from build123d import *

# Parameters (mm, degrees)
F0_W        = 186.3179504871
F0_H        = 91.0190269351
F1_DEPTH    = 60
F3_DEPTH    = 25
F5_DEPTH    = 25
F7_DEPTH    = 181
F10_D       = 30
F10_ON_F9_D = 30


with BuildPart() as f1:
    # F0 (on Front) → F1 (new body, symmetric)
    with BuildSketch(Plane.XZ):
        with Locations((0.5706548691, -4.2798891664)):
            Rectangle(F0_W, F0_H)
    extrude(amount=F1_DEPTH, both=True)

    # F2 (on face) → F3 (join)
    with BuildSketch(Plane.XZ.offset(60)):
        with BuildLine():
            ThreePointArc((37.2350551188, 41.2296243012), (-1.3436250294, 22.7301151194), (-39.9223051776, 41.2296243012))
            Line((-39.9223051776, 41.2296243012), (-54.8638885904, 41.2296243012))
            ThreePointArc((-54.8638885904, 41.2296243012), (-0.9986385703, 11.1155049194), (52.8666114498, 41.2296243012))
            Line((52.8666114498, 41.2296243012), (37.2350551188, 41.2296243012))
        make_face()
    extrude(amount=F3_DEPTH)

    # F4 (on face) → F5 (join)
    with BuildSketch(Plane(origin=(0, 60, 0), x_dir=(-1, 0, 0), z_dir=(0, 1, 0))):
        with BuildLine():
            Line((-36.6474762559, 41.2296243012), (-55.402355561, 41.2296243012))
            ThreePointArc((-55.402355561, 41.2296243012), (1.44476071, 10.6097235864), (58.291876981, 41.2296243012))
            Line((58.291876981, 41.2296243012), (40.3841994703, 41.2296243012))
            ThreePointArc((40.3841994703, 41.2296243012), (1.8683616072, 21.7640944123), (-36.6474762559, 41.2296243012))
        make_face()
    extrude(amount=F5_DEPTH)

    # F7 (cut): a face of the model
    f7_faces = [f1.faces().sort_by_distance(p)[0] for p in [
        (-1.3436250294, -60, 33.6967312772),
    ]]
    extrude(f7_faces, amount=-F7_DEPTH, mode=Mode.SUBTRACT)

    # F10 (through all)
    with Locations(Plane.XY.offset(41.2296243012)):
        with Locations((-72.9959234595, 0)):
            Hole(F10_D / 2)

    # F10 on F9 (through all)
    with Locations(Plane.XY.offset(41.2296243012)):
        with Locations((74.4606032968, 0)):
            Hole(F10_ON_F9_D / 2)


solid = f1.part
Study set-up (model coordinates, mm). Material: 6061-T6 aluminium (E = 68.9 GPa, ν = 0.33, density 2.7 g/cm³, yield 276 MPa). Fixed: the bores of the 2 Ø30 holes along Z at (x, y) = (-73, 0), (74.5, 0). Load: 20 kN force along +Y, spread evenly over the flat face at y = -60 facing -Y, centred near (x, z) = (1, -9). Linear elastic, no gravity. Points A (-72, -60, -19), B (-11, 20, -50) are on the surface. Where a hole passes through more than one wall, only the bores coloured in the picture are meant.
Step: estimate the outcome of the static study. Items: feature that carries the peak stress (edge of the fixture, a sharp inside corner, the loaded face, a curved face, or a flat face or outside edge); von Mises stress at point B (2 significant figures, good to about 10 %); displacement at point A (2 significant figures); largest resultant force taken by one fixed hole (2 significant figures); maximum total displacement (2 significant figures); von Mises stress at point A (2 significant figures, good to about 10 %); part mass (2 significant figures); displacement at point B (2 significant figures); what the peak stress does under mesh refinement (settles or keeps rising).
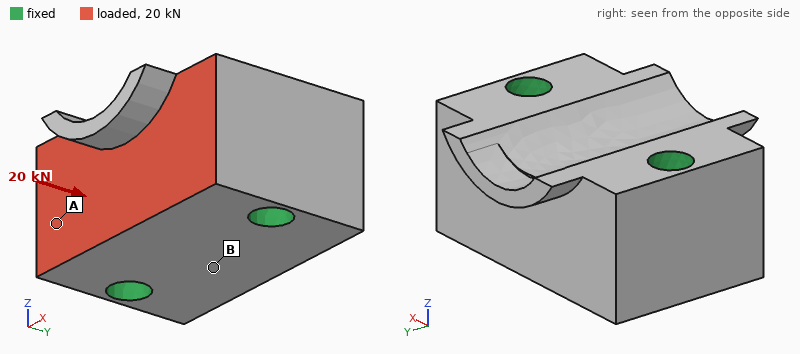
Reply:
edge of the fixture
0.57 MPa
1.1 µm
10 kN
2.6 µm
1.5 MPa
5.0 kg
1.4 µm
keeps rising
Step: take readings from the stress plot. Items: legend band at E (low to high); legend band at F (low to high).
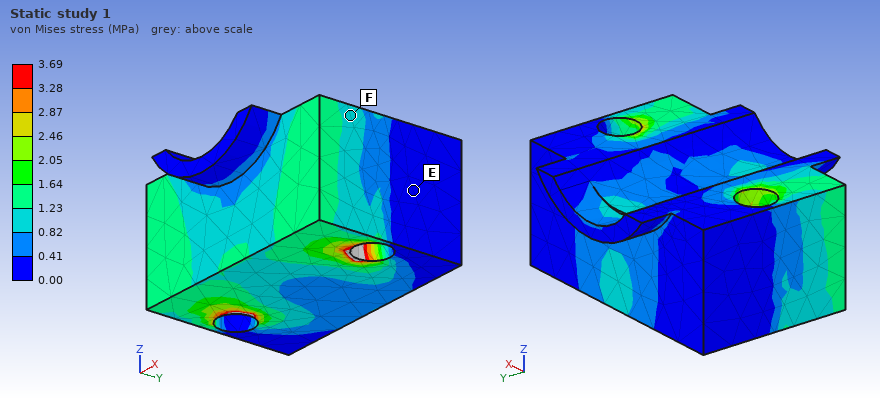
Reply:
0.00 to 0.41 MPa
0.82 to 1.23 MPa
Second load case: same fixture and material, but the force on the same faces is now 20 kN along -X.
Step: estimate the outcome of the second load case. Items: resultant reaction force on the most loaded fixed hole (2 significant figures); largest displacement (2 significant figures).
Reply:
12 kN
5.3 µm
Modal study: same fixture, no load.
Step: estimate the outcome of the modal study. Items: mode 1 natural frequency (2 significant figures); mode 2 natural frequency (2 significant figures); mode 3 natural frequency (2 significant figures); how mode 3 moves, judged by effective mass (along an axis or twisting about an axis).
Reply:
7600 Hz
7800 Hz
8900 Hz
along Y
